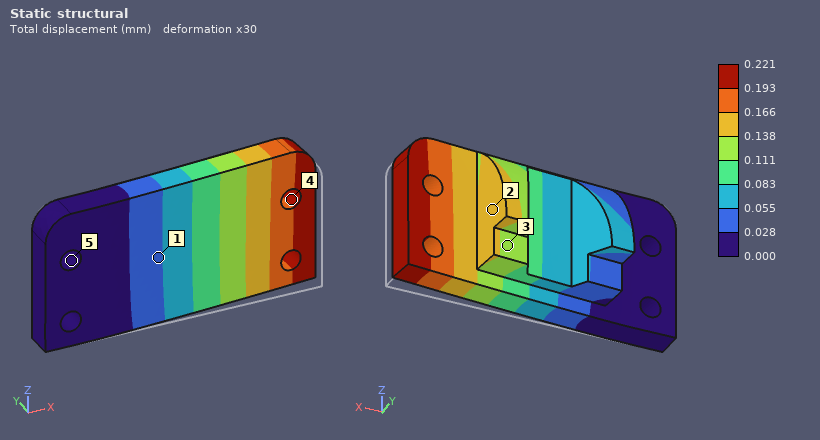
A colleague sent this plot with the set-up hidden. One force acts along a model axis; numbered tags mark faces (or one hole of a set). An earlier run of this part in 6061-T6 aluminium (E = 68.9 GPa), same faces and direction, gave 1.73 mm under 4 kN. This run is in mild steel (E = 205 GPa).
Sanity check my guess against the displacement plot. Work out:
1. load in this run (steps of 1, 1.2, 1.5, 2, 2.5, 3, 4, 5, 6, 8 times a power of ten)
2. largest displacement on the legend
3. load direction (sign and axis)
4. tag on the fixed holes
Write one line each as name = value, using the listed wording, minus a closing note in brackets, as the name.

load in this run = 1.5 kN
largest displacement on the legend = 0.221 mm
load direction = +Y
tag on the fixed holes = 5
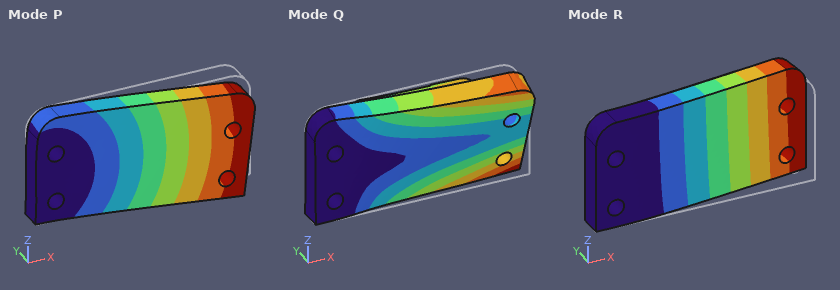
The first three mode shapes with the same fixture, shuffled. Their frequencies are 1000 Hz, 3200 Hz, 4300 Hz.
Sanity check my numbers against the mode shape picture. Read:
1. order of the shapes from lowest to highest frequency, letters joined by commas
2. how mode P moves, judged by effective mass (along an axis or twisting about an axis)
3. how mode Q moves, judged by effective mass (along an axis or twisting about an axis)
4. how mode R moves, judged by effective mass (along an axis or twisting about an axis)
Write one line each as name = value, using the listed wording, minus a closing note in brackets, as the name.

order of the shapes from lowest to highest frequency, letters joined by commas = R, P, Q
how mode P moves, judged by effective mass = along Z
how mode Q moves, judged by effective mass = twisting about X
how mode R moves, judged by effective mass = along Y
